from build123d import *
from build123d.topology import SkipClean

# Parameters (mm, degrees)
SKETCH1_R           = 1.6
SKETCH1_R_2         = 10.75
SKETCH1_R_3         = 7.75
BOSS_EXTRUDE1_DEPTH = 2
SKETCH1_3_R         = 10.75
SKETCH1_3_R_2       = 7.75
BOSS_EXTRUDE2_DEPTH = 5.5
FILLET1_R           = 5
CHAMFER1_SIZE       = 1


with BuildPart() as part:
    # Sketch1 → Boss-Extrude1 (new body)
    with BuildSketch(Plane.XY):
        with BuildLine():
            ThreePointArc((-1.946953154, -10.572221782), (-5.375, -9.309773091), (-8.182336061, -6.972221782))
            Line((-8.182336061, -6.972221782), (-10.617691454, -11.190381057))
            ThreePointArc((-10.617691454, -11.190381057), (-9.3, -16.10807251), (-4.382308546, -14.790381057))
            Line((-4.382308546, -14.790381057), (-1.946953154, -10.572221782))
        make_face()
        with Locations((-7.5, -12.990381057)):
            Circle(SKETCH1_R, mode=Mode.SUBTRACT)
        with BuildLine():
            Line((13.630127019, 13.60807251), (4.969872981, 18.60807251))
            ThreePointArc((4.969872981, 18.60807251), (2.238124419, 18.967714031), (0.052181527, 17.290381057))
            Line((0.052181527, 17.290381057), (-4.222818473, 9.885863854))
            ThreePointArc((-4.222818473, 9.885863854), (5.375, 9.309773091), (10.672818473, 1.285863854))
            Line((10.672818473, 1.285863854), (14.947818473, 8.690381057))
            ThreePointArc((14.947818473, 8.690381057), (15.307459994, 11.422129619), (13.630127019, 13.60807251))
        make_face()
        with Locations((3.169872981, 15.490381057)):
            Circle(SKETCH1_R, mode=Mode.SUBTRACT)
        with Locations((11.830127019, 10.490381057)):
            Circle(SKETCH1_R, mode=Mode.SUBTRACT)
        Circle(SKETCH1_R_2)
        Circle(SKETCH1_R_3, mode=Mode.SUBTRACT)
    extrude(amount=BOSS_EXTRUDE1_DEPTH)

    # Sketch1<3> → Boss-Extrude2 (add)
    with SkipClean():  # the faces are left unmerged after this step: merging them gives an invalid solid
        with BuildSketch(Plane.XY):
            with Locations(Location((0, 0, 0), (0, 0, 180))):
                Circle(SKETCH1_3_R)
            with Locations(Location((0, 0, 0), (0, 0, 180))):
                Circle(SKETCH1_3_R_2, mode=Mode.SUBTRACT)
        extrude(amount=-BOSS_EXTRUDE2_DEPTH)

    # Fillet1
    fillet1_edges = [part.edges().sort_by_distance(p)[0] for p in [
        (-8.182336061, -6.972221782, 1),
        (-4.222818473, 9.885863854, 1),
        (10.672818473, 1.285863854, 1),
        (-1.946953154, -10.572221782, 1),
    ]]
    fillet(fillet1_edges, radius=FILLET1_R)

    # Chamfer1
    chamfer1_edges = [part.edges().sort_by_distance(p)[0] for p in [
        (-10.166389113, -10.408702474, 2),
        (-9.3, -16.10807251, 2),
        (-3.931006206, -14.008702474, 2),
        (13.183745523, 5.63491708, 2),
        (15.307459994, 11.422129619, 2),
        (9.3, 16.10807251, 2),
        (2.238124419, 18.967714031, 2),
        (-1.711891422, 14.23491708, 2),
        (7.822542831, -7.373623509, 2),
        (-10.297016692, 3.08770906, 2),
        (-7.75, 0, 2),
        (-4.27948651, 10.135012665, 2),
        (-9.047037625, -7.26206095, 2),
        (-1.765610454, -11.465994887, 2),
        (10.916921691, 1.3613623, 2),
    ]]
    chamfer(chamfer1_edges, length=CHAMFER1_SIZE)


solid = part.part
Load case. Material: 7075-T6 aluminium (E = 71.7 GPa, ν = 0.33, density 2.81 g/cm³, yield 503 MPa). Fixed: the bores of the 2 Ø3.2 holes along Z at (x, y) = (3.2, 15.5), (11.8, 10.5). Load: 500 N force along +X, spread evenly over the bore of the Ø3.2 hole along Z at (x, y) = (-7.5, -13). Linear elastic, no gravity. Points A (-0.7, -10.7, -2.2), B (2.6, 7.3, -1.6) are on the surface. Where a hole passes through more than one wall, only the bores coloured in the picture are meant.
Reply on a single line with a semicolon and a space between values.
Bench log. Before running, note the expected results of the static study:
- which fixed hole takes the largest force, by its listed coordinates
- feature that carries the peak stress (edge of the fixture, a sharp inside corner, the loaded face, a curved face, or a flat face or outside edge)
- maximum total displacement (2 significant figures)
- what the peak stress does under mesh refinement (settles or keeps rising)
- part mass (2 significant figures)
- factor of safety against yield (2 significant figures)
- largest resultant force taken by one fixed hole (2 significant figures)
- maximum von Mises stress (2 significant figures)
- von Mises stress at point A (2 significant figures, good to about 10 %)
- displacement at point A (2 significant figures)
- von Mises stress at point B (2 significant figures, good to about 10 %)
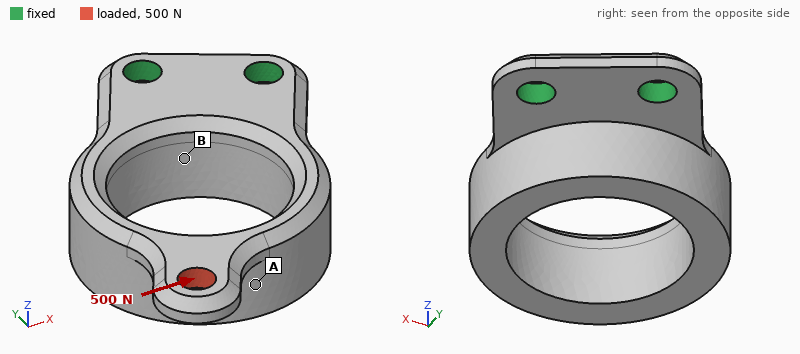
(11.8, 10.5); a curved face; 0.24 mm; settles; 4.5 g; 1.1; 1.2 kN; 460 MPa; 42 MPa; 0.16 mm; 90 MPa
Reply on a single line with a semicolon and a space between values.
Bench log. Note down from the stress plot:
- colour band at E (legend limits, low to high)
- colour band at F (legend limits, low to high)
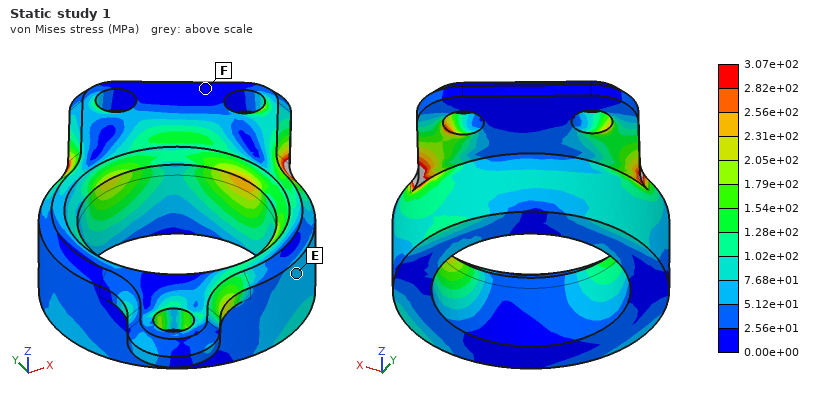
5.12e+01 to 7.68e+01 MPa; 0.00e+00 to 2.56e+01 MPa
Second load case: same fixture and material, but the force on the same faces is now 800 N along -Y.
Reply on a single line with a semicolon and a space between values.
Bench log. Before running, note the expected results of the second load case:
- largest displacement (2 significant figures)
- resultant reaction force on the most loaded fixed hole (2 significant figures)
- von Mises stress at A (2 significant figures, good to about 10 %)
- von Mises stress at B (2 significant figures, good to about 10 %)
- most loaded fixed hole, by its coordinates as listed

0.26 mm; 1.3 kN; 58 MPa; 120 MPa; (3.2, 15.5)
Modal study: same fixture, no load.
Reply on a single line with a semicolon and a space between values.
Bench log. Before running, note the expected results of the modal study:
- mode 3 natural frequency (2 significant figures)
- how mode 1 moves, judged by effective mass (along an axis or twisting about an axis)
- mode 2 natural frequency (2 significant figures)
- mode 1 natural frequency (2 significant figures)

8500 Hz; along Z; 6300 Hz; 2100 Hz
